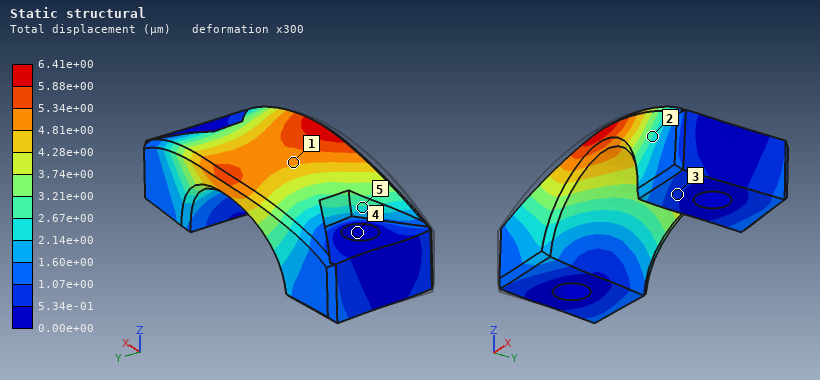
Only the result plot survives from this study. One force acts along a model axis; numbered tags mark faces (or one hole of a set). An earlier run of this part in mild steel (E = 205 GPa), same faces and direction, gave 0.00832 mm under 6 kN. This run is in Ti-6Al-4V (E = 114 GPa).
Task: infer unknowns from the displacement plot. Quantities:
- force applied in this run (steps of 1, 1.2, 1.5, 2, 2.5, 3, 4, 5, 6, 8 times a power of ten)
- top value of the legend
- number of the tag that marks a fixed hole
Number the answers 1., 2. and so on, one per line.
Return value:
1. 2.5 kN
2. 6.41e+00 µm
3. 4
